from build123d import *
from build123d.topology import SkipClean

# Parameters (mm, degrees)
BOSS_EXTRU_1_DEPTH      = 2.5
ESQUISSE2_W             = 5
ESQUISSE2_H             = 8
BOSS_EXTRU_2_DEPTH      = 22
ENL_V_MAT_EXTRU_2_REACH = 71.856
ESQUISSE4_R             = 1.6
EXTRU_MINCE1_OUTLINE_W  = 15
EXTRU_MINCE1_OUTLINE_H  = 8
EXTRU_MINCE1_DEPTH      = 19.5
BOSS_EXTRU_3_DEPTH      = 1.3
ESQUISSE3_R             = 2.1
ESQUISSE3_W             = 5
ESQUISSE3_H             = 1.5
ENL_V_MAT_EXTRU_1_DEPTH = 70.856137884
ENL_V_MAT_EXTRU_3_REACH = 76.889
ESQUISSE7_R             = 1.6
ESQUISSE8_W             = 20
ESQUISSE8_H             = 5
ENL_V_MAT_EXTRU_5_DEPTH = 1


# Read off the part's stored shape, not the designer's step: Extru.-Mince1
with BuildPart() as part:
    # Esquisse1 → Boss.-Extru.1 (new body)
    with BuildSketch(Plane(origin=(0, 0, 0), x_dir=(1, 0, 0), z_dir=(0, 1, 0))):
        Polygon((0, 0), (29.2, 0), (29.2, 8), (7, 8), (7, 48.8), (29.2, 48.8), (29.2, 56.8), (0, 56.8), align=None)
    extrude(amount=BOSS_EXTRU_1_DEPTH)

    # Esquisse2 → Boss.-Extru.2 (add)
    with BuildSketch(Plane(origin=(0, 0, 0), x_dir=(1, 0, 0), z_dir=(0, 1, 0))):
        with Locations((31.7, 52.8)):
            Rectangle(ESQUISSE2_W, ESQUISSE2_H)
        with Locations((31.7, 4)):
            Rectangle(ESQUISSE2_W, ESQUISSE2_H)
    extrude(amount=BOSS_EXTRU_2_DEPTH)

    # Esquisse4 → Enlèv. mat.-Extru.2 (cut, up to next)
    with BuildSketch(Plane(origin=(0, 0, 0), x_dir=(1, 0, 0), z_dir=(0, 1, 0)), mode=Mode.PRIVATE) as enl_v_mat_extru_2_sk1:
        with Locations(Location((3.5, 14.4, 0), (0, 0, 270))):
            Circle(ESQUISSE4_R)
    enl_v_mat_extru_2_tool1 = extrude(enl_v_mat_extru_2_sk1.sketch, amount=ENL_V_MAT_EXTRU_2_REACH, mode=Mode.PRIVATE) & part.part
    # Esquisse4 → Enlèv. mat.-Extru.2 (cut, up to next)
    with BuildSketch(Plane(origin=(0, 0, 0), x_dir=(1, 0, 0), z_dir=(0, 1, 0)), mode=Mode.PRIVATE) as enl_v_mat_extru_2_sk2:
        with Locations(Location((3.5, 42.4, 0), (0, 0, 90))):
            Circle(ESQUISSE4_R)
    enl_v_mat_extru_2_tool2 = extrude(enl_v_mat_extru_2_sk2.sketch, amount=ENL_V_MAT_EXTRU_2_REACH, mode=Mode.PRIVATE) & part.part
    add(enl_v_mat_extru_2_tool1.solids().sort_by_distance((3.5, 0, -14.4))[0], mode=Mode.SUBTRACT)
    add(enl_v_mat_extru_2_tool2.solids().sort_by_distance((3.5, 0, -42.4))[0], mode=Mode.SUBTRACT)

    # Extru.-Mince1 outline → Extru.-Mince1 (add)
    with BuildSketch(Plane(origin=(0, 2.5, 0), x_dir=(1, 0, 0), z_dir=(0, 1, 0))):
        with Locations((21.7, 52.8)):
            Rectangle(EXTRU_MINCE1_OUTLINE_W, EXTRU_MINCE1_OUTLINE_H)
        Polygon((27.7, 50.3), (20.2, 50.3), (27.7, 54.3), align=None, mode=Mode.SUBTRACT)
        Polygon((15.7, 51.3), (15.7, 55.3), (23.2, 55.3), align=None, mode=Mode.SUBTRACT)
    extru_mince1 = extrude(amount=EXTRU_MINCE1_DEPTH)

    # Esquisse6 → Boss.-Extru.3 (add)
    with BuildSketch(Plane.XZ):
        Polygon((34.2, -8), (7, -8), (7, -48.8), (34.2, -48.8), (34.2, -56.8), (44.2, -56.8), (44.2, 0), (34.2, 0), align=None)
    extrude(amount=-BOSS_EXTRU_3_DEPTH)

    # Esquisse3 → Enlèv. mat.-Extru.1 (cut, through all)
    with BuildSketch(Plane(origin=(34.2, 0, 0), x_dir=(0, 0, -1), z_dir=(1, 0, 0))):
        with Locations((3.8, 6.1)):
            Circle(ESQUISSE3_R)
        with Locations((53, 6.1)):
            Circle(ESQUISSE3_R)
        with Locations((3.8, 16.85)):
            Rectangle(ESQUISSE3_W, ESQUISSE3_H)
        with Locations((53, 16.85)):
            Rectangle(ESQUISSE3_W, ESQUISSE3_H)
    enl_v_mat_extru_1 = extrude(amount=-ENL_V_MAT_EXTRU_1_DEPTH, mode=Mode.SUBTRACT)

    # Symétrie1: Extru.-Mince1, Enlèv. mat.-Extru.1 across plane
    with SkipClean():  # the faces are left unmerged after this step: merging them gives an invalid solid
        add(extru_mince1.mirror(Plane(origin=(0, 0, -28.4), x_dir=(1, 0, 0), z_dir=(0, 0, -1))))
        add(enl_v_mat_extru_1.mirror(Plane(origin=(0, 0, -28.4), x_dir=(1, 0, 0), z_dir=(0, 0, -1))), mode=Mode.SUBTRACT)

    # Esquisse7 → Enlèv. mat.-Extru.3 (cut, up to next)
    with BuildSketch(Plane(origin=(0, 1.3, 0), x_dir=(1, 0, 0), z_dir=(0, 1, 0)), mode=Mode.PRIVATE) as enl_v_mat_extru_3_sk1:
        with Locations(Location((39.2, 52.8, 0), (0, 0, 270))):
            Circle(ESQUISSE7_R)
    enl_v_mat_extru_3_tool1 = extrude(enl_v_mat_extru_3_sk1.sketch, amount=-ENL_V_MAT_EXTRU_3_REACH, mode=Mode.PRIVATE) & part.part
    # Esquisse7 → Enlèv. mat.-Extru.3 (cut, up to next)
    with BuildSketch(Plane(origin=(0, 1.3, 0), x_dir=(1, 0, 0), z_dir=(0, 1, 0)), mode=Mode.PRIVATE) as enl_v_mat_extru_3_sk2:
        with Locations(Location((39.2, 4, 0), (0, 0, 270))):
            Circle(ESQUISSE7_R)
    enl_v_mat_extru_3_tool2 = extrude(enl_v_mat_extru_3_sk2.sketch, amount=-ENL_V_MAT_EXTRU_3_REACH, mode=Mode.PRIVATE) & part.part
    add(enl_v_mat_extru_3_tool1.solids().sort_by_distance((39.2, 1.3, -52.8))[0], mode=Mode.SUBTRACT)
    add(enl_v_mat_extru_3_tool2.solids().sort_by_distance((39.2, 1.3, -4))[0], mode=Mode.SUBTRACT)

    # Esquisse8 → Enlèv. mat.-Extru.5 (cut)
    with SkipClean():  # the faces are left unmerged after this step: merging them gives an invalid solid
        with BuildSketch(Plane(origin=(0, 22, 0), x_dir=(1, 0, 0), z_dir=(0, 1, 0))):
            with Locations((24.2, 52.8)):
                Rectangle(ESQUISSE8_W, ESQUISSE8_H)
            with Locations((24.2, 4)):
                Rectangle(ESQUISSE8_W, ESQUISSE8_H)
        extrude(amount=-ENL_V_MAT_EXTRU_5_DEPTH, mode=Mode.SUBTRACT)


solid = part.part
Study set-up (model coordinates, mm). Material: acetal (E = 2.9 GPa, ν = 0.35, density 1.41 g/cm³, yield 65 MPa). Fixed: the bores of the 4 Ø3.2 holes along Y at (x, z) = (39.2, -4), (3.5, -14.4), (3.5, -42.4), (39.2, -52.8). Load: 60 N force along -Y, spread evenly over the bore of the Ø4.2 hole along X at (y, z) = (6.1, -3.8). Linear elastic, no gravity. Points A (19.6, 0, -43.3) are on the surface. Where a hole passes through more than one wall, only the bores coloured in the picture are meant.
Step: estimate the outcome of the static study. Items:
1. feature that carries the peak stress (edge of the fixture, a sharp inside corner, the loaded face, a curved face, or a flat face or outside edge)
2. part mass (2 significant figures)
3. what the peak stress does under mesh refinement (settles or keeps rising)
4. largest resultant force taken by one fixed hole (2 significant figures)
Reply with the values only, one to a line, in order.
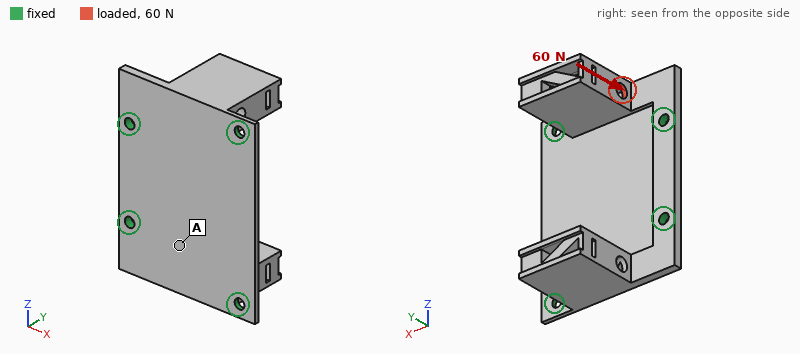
edge of the fixture
12 g
keeps rising
34 N
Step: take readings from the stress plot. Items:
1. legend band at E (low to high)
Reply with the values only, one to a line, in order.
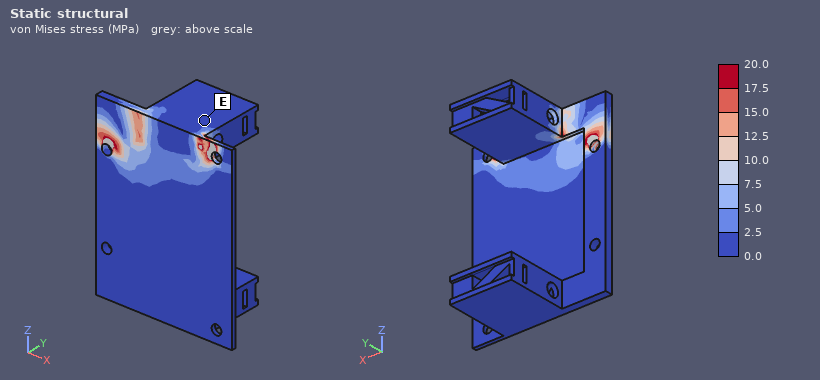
0.0 to 2.5 MPa
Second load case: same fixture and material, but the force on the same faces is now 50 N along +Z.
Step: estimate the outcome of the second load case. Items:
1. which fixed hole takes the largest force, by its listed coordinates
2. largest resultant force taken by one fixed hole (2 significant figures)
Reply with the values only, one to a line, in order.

(3.5, -14.4)
21 N
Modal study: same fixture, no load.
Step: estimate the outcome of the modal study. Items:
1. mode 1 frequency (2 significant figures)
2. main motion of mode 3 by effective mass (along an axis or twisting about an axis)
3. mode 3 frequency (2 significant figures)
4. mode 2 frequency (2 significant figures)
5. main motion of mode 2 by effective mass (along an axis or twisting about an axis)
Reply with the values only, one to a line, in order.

550 Hz
along Y
1100 Hz
600 Hz
along Z
